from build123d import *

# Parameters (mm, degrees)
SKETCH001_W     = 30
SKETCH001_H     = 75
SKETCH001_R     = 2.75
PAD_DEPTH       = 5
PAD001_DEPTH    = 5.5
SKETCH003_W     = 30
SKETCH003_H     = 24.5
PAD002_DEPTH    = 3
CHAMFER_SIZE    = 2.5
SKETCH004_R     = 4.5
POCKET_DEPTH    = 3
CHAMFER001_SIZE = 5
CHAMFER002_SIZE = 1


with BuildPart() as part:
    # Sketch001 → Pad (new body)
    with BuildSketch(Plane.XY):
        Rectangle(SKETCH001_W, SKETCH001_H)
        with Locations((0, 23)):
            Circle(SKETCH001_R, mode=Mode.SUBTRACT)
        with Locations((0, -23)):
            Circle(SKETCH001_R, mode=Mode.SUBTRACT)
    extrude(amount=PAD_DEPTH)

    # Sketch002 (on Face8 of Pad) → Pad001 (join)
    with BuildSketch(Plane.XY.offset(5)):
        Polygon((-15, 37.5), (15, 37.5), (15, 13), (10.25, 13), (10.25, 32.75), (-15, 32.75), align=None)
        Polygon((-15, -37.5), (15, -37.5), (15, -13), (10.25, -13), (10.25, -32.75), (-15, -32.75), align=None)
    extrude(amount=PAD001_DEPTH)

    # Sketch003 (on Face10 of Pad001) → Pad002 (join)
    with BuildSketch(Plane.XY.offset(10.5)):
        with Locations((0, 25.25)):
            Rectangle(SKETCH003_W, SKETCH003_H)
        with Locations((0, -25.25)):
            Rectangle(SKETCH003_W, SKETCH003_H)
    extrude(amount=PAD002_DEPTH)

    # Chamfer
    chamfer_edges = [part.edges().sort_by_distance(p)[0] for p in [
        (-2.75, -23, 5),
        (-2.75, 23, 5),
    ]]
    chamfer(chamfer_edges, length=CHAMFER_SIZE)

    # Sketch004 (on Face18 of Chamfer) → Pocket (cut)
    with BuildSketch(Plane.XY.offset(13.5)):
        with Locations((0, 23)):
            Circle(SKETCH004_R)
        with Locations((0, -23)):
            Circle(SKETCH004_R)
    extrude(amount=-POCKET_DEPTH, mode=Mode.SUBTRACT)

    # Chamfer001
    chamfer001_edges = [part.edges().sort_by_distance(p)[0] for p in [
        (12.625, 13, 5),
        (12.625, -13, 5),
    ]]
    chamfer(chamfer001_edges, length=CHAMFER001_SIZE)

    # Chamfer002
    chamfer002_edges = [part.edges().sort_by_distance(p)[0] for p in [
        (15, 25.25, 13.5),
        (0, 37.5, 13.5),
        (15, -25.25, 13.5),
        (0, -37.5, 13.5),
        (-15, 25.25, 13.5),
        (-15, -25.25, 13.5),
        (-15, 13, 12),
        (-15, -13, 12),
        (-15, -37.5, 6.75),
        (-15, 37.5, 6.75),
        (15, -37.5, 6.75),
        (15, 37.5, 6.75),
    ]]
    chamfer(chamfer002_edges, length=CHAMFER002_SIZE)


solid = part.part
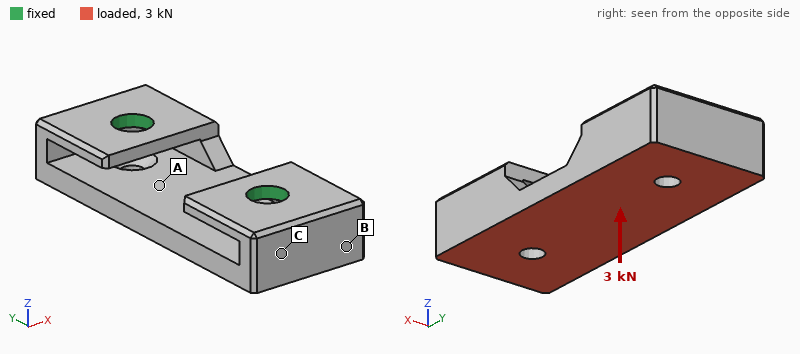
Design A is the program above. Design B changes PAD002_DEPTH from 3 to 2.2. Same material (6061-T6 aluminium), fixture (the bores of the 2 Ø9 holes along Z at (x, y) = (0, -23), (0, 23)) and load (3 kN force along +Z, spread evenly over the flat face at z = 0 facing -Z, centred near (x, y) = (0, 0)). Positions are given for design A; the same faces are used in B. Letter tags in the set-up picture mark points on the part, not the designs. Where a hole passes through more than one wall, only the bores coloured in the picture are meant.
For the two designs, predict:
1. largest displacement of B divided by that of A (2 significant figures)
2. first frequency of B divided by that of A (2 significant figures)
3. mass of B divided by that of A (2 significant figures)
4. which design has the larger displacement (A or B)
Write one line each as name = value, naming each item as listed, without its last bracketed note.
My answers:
largest displacement of B divided by that of A = 1.3
first frequency of B divided by that of A = 0.78
mass of B divided by that of A = 0.94
which design has the larger displacement = B
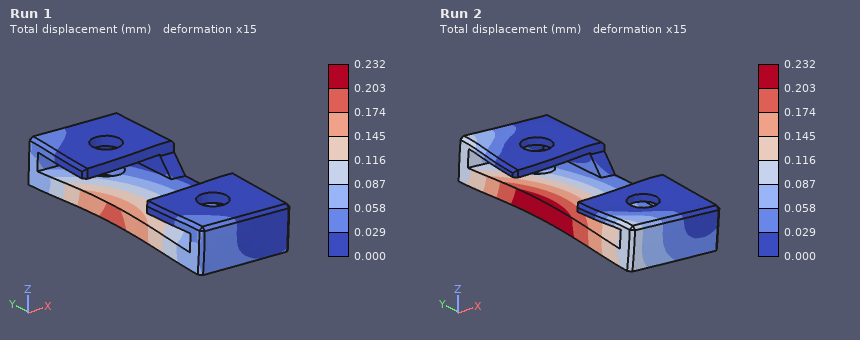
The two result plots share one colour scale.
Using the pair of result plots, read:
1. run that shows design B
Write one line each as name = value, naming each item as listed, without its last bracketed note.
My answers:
run that shows design B = Run 2
